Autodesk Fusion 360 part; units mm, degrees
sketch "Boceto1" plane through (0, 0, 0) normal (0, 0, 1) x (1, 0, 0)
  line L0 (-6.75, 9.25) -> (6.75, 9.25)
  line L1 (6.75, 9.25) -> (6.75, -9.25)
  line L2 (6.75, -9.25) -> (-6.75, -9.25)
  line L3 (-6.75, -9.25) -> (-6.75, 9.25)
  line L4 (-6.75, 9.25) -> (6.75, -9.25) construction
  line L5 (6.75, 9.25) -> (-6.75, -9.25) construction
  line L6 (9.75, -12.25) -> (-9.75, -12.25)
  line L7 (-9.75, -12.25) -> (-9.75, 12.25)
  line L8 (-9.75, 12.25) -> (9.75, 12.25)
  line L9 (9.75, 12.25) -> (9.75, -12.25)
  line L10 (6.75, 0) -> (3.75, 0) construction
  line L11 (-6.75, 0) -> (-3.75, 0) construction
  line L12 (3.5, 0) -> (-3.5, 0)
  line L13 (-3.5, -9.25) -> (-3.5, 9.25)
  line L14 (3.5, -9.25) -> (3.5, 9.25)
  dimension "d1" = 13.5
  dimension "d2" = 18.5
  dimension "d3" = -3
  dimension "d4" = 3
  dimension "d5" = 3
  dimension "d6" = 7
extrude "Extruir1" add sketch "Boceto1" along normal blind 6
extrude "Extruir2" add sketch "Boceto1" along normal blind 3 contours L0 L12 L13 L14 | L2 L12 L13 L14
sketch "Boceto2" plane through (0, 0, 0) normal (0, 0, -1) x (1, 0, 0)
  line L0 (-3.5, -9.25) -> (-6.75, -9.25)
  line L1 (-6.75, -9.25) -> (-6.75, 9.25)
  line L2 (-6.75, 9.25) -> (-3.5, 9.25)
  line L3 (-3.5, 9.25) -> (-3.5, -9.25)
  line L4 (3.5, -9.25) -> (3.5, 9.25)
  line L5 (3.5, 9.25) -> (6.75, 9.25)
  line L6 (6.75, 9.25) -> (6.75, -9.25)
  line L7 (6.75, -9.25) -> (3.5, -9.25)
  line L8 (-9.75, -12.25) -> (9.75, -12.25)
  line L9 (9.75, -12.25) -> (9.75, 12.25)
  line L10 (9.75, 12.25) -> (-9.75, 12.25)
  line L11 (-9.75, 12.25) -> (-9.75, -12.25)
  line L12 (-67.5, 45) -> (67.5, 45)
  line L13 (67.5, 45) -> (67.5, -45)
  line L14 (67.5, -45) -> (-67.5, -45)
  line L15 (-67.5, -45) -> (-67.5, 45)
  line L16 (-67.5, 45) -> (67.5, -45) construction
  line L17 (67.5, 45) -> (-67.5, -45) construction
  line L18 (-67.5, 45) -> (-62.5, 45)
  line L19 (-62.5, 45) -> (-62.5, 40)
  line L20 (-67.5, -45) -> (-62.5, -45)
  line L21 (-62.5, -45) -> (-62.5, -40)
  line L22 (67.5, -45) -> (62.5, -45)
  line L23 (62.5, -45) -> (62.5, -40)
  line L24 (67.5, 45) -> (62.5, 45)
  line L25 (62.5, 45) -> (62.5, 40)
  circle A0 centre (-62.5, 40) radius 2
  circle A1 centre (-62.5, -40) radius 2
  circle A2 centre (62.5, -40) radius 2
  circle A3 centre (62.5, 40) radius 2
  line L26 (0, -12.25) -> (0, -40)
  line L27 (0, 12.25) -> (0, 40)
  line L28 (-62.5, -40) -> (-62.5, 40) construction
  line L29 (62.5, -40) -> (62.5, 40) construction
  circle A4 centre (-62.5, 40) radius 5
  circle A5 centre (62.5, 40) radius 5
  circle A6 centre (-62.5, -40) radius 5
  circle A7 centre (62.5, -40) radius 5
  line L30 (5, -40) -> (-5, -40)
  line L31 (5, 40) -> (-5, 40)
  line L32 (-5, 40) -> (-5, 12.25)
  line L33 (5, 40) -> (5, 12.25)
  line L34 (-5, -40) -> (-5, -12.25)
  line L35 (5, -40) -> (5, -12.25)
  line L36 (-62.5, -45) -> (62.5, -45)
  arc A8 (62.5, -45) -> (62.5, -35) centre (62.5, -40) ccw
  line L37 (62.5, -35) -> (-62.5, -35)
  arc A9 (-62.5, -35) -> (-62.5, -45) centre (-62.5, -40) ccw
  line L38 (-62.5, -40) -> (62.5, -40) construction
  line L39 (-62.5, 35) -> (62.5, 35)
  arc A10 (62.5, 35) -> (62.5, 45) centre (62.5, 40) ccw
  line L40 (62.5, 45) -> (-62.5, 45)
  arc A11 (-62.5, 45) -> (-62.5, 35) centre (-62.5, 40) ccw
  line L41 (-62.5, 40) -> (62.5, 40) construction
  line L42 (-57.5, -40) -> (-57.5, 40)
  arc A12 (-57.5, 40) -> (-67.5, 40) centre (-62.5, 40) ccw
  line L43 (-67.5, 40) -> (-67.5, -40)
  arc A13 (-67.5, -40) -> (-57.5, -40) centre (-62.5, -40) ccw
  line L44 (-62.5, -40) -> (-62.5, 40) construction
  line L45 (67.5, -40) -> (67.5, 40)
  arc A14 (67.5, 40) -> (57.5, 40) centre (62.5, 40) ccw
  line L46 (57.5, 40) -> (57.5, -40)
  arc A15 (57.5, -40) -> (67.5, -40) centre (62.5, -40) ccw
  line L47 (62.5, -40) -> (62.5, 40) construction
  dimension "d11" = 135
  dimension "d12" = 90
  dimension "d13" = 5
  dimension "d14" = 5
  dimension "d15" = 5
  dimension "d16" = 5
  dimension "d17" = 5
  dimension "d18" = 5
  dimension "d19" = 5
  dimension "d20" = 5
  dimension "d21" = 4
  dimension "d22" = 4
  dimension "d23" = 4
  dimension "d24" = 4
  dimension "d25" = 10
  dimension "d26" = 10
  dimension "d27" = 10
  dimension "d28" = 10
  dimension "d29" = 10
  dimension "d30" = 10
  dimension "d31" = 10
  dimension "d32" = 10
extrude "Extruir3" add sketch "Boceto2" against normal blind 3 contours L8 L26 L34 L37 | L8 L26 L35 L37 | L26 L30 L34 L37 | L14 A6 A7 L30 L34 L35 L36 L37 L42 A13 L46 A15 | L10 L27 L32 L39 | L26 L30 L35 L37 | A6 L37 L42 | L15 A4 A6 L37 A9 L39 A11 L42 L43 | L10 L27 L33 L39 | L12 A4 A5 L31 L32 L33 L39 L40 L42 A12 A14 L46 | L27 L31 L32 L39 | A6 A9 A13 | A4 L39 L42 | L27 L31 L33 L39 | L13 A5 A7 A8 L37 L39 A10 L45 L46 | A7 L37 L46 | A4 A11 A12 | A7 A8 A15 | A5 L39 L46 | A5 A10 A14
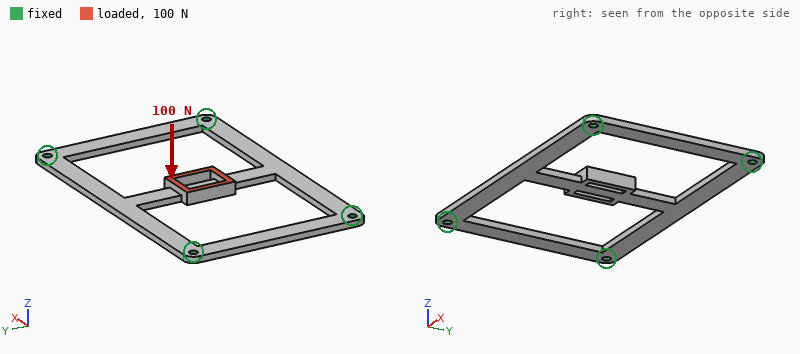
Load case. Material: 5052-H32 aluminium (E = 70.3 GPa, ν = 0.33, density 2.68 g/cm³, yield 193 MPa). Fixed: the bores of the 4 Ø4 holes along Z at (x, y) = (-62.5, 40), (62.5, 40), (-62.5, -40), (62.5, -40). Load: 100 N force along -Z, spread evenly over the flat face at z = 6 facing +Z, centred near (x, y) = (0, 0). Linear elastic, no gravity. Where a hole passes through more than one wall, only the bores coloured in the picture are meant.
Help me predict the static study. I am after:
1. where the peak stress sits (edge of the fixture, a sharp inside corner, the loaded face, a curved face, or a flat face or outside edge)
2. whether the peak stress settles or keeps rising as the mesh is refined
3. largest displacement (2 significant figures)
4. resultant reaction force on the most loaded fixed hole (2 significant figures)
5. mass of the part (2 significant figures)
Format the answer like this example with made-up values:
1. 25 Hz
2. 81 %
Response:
1. edge of the fixture
2. keeps rising
3. 0.49 mm
4. 25 N
5. 41 g
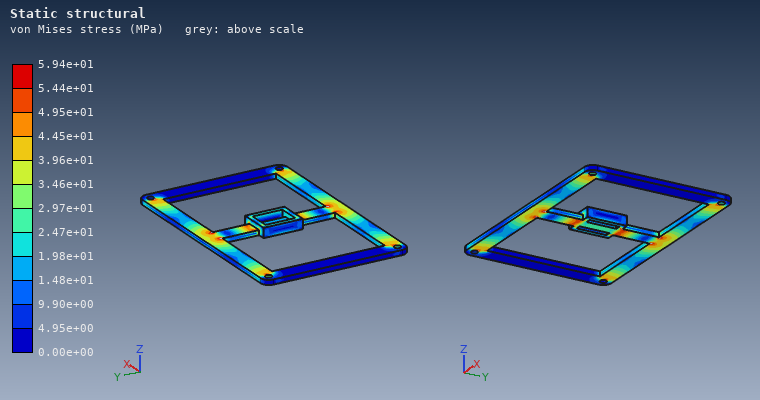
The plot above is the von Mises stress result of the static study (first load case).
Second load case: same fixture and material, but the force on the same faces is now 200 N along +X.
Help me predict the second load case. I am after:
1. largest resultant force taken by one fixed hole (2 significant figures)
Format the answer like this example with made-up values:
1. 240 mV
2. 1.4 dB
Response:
1. 52 N
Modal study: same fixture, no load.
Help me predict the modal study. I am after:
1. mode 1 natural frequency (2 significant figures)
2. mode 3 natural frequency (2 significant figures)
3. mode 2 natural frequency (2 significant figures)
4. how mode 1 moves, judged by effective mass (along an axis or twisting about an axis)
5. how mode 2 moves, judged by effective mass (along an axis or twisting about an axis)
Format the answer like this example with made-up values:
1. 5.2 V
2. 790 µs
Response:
1. 690 Hz
2. 2100 Hz
3. 1000 Hz
4. along Z
5. twisting about X
